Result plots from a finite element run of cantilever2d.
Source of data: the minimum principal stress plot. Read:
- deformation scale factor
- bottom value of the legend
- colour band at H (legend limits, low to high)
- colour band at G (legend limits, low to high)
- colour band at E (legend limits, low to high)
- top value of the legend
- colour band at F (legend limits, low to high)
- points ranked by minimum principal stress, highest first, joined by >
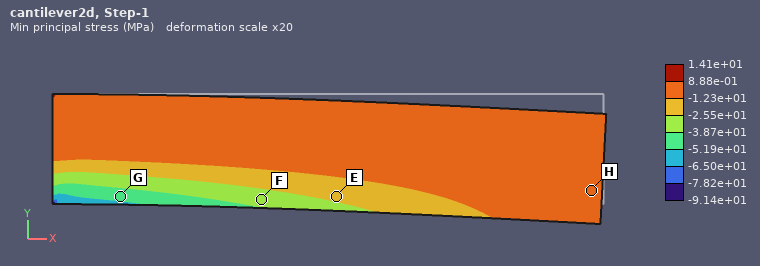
20
-9.14e+01 MPa
-1.23e+01 to 8.88e-01 MPa
-5.19e+01 to -3.87e+01 MPa
-2.55e+01 to -1.23e+01 MPa
1.41e+01 MPa
-3.87e+01 to -2.55e+01 MPa
H > E > F > G
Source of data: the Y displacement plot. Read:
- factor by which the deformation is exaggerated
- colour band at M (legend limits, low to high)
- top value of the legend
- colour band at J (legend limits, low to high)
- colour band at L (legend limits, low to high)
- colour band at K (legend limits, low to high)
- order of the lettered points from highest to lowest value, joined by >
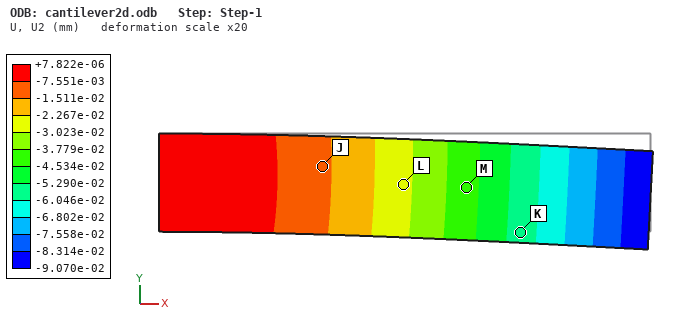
20
-4.534e-02 to -3.779e-02 mm
+7.822e-06 mm
-1.511e-02 to -7.551e-03 mm
-3.023e-02 to -2.267e-02 mm
-6.046e-02 to -5.290e-02 mm
J > L > M > K
